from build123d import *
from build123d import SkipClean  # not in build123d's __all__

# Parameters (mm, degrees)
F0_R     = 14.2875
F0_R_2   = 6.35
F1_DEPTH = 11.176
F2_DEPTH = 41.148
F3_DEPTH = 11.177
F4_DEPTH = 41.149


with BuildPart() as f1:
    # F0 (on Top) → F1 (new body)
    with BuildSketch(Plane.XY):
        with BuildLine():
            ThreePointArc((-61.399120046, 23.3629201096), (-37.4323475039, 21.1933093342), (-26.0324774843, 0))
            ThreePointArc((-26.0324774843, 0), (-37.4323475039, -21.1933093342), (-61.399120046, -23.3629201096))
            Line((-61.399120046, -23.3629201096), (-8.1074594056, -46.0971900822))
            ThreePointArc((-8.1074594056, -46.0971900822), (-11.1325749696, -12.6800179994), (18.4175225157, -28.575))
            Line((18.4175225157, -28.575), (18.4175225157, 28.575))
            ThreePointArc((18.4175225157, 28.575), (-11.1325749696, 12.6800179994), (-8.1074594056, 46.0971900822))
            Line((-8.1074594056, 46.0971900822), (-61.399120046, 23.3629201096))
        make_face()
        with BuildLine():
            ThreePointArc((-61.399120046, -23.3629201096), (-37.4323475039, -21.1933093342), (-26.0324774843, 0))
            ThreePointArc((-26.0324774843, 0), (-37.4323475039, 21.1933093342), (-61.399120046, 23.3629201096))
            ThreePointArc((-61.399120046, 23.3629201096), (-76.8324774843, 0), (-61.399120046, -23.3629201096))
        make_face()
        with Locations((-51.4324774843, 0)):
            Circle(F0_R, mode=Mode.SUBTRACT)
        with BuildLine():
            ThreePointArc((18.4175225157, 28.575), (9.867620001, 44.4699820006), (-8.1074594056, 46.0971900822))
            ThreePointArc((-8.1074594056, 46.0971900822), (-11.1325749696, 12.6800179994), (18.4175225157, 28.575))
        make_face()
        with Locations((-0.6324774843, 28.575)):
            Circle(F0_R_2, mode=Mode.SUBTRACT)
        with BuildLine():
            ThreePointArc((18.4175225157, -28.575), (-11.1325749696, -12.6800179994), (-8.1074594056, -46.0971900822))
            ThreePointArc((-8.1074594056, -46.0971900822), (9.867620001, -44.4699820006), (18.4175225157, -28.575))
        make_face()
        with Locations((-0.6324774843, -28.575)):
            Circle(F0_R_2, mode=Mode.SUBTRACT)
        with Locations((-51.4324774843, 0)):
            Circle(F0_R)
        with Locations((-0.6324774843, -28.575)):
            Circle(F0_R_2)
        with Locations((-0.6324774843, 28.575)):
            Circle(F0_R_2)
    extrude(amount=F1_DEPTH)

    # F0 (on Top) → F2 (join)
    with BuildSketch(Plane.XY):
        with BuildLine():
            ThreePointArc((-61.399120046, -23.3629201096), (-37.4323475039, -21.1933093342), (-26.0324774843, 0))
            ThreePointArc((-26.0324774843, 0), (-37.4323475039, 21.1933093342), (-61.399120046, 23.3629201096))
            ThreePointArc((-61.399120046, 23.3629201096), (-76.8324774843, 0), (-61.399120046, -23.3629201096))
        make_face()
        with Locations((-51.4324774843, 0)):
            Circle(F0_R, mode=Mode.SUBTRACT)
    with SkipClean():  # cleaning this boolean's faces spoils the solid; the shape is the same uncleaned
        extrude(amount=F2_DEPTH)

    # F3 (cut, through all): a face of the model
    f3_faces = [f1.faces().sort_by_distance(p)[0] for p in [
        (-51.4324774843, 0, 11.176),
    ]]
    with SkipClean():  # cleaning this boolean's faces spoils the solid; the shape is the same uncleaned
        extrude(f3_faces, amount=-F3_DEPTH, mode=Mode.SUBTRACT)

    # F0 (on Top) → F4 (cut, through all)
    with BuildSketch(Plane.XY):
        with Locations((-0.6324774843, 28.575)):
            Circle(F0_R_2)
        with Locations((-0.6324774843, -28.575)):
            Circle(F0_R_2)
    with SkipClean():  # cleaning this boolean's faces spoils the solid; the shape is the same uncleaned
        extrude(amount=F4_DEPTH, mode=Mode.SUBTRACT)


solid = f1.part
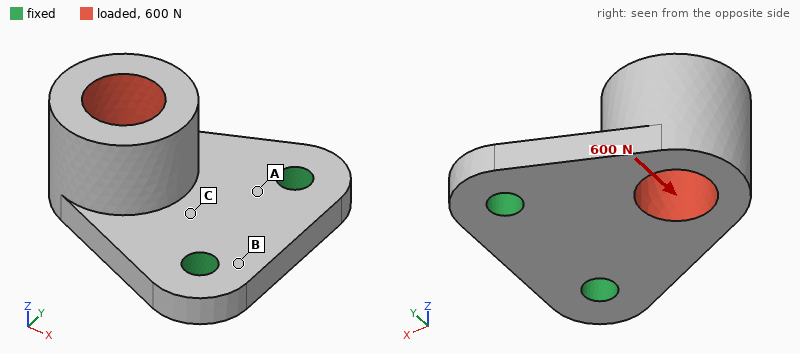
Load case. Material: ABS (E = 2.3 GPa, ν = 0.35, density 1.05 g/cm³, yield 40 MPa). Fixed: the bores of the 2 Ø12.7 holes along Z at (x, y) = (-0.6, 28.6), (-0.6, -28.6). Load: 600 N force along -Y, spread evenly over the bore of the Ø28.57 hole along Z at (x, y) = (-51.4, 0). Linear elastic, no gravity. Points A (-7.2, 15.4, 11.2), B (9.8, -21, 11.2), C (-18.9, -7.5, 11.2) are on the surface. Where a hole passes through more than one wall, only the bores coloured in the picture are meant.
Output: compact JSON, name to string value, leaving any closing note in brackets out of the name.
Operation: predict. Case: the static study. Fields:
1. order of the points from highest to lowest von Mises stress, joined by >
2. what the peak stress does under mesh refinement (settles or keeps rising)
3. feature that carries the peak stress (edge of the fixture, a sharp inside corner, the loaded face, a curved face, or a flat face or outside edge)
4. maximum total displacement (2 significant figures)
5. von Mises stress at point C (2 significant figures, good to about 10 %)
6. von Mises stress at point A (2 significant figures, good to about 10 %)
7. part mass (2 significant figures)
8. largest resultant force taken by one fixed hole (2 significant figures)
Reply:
{"order of the points from highest to lowest von Mises stress, joined by >": "C > A > B", "what the peak stress does under mesh refinement": "keeps rising", "feature that carries the peak stress": "edge of the fixture", "maximum total displacement": "0.25 mm", "von Mises stress at point C": "3.3 MPa", "von Mises stress at point A": "2.0 MPa", "part mass": "110 g", "largest resultant force taken by one fixed hole": "570 N"}
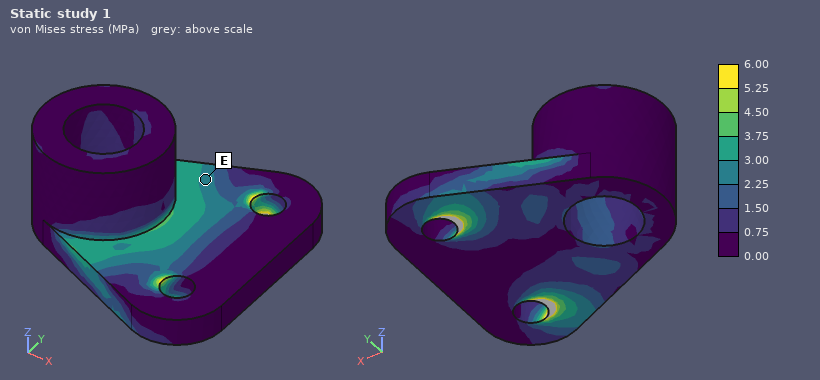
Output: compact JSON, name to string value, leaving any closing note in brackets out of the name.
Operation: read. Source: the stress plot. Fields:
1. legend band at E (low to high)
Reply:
{"legend band at E": "2.25 to 3.00 MPa"}
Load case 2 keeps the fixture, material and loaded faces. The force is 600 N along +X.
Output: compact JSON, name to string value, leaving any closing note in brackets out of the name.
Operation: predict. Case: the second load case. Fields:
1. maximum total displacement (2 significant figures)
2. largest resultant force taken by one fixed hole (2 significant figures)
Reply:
{"maximum total displacement": "0.97 mm", "largest resultant force taken by one fixed hole": "320 N"}
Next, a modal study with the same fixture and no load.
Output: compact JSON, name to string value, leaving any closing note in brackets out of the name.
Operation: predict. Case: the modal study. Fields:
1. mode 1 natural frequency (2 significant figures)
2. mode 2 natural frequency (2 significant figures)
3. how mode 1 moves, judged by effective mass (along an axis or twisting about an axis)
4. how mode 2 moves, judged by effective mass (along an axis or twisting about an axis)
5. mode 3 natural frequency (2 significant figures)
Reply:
{"mode 1 natural frequency": "390 Hz", "mode 2 natural frequency": "1100 Hz", "how mode 1 moves, judged by effective mass": "along Z", "how mode 2 moves, judged by effective mass": "along Y", "mode 3 natural frequency": "1900 Hz"}
